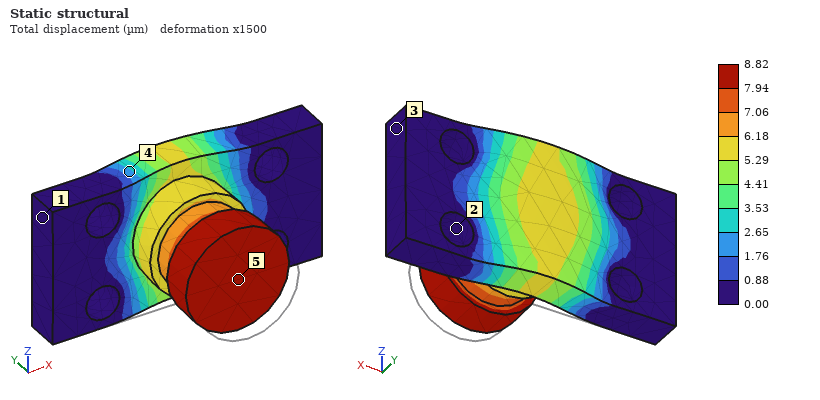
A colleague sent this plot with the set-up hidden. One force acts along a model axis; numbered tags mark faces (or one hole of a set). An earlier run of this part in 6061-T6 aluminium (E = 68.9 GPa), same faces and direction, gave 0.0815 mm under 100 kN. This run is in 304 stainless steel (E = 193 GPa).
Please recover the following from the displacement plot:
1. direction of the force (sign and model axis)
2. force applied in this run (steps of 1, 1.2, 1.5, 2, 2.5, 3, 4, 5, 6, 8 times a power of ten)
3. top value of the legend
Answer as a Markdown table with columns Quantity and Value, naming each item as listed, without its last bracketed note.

| Quantity | Value |
|---|---|
| direction of the force | +Y |
| force applied in this run | 30 kN |
| top value of the legend | 8.82 µm |
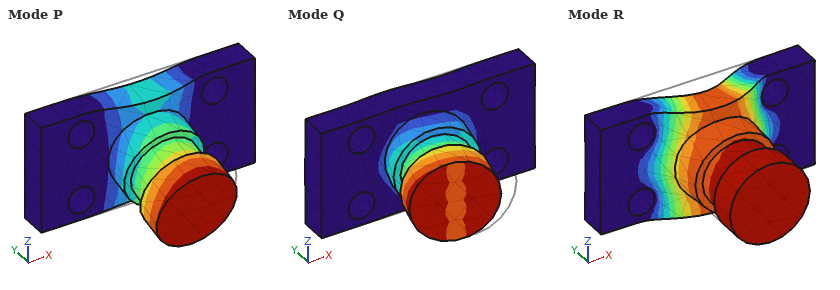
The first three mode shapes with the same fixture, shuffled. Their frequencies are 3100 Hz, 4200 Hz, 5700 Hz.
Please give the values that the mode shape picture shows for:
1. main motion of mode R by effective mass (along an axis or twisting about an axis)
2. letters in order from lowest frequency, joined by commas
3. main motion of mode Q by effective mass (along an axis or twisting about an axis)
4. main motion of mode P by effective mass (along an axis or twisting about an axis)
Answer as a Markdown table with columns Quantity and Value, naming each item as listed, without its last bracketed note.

| Quantity | Value |
|---|---|
| main motion of mode R by effective mass | along Y |
| letters in order from lowest frequency, joined by commas | P, Q, R |
| main motion of mode Q by effective mass | along X |
| main motion of mode P by effective mass | along Z |
